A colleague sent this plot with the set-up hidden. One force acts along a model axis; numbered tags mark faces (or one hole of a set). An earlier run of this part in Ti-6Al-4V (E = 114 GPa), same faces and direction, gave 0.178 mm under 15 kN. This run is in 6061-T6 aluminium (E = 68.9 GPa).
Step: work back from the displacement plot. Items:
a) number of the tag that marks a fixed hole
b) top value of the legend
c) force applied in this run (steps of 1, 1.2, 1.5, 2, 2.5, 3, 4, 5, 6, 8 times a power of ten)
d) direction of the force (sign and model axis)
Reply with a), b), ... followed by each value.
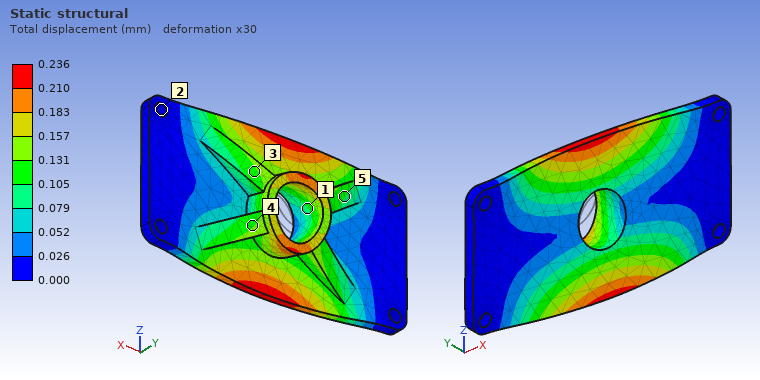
a) 2
b) 0.236 mm
c) 12 kN
d) -Z
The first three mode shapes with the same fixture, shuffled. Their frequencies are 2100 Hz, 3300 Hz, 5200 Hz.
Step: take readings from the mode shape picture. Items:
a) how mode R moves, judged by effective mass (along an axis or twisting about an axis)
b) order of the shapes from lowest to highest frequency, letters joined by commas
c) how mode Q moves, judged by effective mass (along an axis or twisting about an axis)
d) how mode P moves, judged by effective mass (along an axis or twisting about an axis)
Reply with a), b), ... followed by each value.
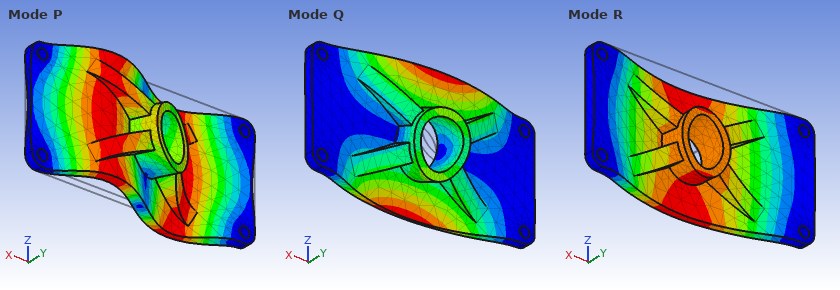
a) along Y
b) R, Q, P
c) twisting about X
d) twisting about Z
